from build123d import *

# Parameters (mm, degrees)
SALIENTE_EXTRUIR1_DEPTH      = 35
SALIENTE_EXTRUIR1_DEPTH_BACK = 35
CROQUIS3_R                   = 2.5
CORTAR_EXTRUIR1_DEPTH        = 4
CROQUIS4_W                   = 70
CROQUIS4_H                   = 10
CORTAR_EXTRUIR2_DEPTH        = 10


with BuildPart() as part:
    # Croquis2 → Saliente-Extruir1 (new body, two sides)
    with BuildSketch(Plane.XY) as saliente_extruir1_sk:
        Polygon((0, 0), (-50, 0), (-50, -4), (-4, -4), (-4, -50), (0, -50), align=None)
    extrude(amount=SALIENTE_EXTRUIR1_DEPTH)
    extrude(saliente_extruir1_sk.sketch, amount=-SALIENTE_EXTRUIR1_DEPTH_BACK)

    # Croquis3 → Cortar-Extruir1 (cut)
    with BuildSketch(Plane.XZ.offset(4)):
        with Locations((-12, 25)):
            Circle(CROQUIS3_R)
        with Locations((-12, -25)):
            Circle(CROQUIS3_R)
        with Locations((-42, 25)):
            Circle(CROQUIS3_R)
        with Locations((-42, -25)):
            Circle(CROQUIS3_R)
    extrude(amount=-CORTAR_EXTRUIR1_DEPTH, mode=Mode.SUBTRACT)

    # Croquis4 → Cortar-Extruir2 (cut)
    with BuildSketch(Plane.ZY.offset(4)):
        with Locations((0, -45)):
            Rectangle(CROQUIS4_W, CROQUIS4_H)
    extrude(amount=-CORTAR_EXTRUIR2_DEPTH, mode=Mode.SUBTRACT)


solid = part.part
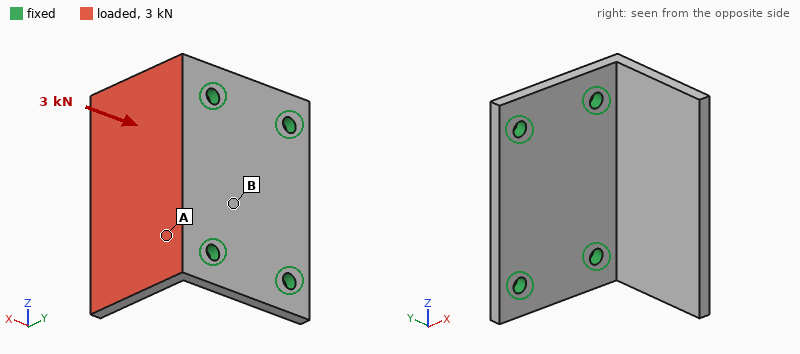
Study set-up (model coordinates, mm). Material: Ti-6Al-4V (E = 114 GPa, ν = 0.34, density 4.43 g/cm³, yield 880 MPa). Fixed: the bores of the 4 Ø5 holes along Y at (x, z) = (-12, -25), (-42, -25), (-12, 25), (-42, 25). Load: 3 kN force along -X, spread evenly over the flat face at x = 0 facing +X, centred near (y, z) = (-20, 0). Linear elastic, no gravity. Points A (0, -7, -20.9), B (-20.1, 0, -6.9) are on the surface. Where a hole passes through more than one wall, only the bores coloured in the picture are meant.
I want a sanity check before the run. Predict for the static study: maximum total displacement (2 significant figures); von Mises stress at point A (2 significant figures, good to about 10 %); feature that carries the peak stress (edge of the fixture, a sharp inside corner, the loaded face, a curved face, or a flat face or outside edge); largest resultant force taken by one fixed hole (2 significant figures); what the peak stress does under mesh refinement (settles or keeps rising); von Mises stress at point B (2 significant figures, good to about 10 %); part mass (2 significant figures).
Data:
0.86 mm
200 MPa
edge of the fixture
1.2 kN
keeps rising
65 MPa
110 g
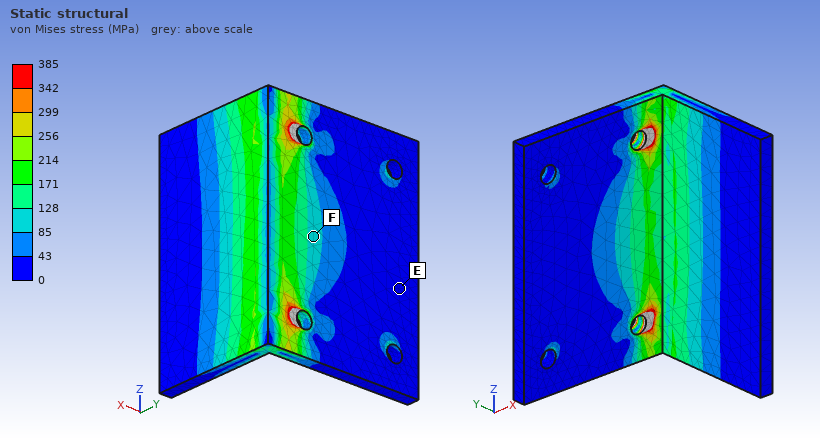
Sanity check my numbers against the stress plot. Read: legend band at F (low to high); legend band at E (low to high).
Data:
85 to 128 MPa
0 to 43 MPa
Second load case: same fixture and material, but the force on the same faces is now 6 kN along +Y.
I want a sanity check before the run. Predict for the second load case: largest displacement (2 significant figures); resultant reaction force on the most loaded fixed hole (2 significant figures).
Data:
0.52 mm
3.3 kN
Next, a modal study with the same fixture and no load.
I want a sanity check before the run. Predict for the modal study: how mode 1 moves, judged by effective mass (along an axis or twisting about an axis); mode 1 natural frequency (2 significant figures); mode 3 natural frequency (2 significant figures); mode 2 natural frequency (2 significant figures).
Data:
along X
1600 Hz
6700 Hz
3000 Hz
